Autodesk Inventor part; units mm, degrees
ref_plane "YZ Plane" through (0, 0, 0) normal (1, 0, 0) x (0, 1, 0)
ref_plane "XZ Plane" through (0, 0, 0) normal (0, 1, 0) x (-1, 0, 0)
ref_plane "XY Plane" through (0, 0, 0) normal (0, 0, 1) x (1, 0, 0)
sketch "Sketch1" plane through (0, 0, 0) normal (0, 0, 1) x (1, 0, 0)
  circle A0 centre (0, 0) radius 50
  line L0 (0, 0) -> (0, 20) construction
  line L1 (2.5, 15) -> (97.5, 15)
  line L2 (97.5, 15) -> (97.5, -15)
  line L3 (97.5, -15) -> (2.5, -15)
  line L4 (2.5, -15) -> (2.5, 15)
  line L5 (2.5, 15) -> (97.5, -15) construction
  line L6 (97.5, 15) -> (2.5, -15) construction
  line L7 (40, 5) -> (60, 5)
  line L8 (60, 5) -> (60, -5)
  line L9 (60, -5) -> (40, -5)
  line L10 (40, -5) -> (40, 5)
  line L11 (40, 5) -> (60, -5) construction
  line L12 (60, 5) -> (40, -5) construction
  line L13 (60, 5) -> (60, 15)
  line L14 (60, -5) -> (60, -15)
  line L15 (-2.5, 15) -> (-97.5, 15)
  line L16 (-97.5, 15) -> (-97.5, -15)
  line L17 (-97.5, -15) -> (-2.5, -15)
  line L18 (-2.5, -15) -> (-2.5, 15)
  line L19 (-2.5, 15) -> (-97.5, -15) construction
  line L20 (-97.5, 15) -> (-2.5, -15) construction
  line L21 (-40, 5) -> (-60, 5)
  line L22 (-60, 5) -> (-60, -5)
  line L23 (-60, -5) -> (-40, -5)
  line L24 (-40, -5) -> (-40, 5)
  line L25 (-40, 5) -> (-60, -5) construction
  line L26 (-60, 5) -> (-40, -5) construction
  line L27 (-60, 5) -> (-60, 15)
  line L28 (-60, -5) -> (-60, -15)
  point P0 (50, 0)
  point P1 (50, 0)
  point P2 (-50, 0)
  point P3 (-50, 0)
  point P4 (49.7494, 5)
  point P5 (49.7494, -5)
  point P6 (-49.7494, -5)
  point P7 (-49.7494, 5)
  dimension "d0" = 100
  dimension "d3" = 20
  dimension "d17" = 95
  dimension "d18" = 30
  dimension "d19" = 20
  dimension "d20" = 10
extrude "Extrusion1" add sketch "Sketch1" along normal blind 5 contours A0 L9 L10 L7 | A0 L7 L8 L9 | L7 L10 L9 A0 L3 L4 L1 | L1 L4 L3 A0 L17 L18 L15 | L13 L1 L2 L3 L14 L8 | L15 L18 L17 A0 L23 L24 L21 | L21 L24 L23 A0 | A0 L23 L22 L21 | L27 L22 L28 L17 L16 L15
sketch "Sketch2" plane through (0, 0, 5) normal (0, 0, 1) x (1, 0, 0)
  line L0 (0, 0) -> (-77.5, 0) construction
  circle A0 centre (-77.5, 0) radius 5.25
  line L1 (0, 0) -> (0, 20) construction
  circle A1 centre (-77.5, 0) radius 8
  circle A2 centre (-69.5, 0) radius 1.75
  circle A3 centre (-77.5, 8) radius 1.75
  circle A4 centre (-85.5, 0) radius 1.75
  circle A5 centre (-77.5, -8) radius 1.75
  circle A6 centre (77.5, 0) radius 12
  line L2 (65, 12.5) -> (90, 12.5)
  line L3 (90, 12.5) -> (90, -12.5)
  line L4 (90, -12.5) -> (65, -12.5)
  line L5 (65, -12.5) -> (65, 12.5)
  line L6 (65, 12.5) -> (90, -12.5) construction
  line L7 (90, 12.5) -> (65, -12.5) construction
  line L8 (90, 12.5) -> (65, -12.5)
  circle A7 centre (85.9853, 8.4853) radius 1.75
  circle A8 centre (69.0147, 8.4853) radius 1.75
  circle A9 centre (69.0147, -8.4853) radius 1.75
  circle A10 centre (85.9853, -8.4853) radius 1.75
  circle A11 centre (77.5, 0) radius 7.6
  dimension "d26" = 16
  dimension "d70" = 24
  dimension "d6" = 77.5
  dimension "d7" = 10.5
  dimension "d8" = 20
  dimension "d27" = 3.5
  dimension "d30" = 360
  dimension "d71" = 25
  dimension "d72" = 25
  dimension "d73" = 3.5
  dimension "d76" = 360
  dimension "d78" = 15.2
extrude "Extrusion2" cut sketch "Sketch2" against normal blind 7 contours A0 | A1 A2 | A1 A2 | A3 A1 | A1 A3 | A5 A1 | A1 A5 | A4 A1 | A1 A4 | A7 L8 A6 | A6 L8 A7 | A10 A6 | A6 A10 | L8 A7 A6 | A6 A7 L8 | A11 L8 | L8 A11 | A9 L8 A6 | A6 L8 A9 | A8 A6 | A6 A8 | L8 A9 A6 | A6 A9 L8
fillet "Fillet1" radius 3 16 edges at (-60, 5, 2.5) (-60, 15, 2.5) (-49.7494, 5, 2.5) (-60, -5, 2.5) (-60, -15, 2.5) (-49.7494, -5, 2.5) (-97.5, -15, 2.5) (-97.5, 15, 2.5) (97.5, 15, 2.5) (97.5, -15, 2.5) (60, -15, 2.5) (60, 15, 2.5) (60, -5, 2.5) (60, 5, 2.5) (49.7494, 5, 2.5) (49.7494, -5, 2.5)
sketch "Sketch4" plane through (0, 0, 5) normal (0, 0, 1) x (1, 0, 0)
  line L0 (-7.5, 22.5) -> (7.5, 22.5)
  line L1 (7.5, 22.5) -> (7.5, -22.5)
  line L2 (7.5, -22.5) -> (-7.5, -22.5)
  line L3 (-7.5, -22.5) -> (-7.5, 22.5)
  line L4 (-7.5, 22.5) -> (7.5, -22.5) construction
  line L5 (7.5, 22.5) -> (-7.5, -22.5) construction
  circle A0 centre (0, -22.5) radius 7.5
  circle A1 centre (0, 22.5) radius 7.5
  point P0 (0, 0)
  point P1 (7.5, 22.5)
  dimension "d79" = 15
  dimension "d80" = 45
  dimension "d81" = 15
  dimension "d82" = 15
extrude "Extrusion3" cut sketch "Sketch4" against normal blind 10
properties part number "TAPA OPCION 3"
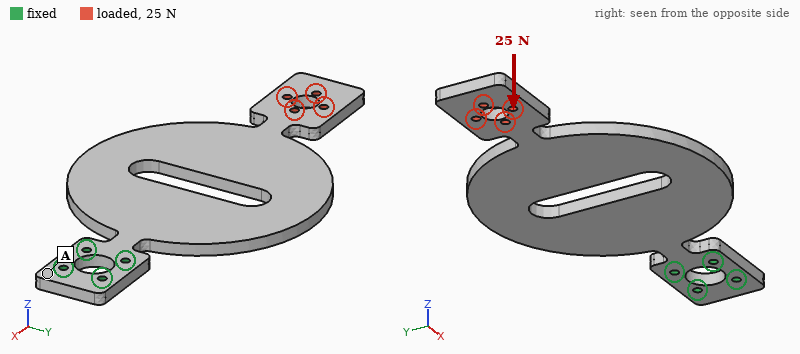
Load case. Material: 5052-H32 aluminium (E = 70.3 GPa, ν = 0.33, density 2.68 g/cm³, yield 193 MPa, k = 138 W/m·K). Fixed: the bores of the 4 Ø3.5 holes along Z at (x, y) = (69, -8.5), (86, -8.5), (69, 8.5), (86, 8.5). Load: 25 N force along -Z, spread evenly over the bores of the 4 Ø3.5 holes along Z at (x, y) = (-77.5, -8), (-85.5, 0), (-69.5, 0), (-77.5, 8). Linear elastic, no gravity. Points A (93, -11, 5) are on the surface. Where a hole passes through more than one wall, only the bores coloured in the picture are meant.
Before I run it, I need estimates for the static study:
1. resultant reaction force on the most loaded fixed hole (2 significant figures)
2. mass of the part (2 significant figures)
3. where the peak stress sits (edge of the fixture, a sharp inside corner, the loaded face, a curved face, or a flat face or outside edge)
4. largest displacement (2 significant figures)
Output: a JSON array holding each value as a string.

["22 N", "120 g", "a curved face", "2.0 mm"]
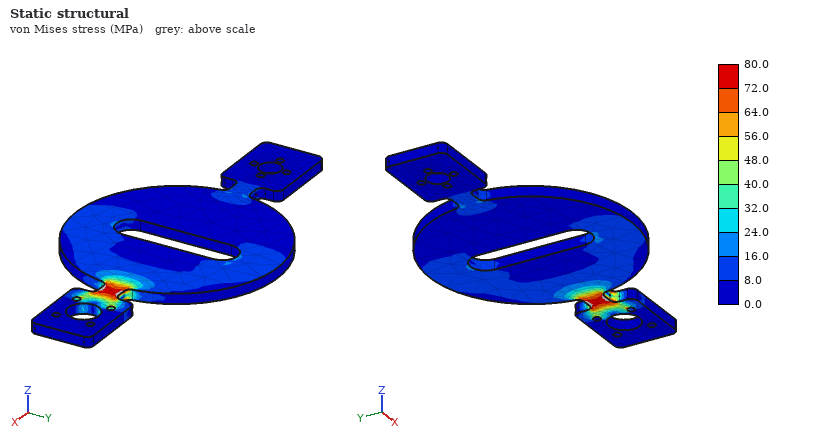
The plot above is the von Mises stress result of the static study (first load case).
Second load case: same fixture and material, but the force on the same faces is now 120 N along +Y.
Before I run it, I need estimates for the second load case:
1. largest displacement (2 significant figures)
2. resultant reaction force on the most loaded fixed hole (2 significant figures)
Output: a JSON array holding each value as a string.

["1.3 mm", "990 N"]
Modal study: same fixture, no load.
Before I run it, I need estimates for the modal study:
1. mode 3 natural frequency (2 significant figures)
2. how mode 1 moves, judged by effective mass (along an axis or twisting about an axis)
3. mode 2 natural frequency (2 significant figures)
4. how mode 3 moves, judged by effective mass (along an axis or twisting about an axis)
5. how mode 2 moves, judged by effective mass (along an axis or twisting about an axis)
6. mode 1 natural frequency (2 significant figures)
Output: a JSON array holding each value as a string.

["390 Hz", "along Z", "270 Hz", "twisting about X", "along Y", "110 Hz"]
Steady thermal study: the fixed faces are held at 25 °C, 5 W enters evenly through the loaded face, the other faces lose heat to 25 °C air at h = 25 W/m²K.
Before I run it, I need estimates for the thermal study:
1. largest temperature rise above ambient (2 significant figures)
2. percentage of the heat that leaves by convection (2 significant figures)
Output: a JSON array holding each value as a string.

["22 K", "78 %"]
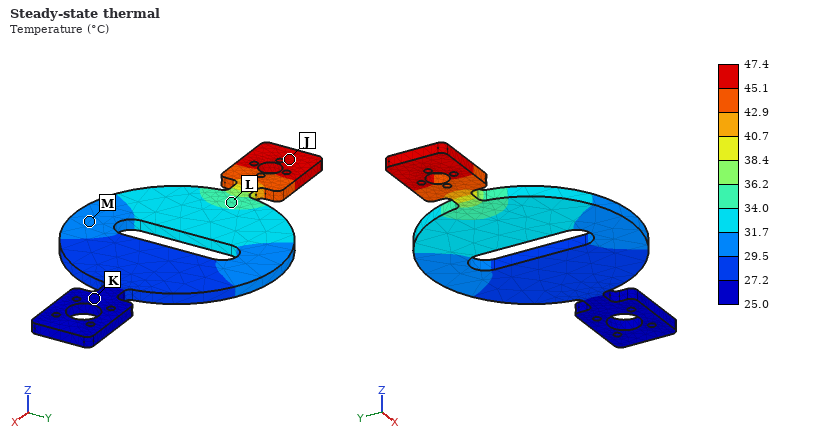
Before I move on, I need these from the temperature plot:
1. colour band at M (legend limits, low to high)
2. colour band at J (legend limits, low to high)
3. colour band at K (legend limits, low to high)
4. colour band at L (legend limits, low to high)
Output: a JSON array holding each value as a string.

["29.5 to 31.7 °C", "45.1 to 47.4 °C", "25.0 to 27.2 °C", "34.0 to 36.2 °C"]
